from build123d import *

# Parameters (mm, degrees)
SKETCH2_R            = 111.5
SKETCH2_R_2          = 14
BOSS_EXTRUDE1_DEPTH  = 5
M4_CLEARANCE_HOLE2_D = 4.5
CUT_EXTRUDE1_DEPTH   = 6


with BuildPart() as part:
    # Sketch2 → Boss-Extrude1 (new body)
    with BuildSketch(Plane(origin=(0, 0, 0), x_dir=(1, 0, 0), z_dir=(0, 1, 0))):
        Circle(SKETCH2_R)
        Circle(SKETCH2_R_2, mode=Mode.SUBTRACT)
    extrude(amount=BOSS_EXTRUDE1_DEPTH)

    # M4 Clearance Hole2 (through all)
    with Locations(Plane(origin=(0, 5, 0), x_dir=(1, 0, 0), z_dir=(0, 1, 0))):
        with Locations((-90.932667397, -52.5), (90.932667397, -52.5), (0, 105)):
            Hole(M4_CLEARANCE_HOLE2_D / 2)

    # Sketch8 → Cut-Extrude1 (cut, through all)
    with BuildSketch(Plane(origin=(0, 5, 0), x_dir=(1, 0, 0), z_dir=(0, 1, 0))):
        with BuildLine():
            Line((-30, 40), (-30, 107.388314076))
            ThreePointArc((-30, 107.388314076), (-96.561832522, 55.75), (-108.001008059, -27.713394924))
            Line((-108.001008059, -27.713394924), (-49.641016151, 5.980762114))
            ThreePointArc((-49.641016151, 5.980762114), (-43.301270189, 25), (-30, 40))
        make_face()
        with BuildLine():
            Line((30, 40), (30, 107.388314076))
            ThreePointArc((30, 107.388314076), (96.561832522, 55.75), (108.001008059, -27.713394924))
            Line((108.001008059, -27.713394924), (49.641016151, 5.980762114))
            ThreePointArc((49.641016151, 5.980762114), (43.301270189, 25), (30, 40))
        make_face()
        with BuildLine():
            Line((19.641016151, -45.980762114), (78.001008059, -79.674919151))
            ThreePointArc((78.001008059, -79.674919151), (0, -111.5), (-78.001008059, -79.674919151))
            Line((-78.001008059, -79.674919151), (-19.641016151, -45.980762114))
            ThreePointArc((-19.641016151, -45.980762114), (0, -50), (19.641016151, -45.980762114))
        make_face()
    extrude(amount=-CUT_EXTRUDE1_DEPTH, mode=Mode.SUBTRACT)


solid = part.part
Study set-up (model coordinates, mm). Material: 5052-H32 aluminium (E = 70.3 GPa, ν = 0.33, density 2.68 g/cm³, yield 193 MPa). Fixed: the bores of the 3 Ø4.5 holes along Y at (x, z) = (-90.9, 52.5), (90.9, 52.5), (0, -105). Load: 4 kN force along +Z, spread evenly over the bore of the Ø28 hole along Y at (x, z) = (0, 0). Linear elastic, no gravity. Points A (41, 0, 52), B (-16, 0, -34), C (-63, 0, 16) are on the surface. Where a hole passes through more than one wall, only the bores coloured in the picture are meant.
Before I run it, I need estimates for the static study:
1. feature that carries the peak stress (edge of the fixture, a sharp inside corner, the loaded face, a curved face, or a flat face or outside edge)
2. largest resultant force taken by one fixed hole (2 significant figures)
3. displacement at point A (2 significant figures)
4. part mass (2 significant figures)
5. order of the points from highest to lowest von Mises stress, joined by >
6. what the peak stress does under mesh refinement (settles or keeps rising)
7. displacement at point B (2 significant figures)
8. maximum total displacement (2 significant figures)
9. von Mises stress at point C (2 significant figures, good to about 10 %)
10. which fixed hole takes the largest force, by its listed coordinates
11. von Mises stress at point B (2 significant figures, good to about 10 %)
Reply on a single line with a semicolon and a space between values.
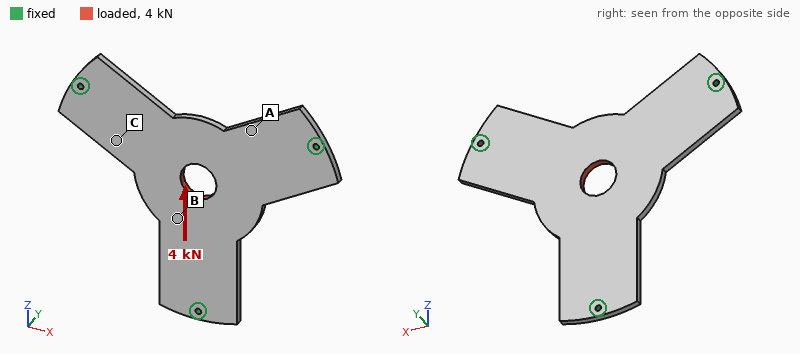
edge of the fixture; 2.4 kN; 15 µm; 250 g; B > C > A; keeps rising; 14 µm; 24 µm; 6.0 MPa; (0, -105); 9.6 MPa
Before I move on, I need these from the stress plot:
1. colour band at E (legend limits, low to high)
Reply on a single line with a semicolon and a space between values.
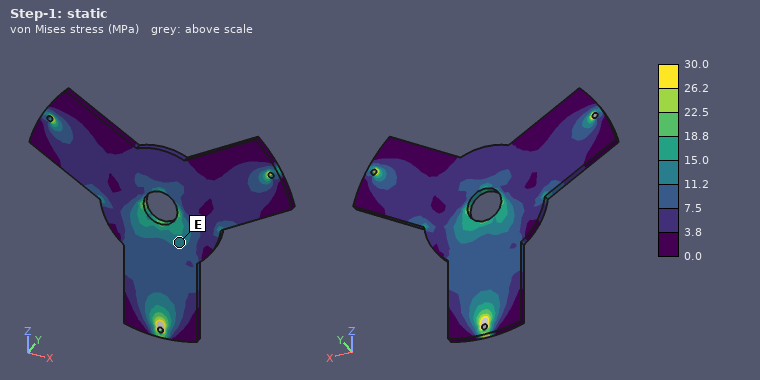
11.2 to 15.0 MPa
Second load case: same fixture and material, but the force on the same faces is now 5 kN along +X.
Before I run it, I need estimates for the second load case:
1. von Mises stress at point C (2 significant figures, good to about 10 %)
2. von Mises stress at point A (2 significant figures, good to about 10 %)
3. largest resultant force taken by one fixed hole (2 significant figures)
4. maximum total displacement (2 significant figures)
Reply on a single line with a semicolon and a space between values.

7.7 MPa; 10 MPa; 2.6 kN; 30 µm
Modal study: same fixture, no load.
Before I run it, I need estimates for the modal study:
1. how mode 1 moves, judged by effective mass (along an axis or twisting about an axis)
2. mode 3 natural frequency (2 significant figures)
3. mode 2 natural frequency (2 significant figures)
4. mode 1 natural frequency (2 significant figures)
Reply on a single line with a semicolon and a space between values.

along Y; 1300 Hz; 1300 Hz; 630 Hz
